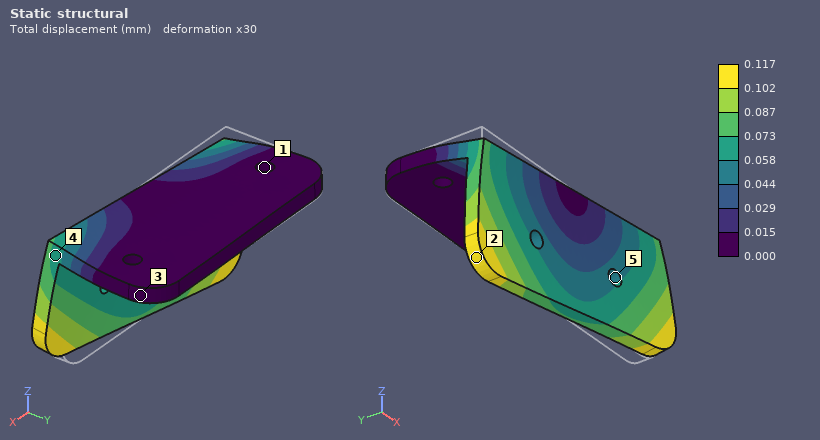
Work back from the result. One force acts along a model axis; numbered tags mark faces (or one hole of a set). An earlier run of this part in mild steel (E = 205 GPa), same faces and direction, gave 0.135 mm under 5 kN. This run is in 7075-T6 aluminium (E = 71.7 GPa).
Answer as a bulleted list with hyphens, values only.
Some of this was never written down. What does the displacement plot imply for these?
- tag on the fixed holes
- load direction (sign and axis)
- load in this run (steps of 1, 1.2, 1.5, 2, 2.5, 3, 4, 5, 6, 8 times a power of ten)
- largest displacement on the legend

- 1
- +X
- 1.5 kN
- 0.117 mm
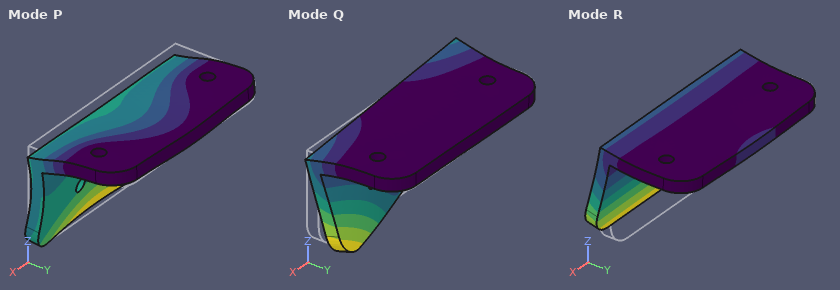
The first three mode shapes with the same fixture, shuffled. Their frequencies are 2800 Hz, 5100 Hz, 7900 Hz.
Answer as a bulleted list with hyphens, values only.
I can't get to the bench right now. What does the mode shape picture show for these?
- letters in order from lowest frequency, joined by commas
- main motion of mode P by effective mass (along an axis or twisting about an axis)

- R, Q, P
- along Z
